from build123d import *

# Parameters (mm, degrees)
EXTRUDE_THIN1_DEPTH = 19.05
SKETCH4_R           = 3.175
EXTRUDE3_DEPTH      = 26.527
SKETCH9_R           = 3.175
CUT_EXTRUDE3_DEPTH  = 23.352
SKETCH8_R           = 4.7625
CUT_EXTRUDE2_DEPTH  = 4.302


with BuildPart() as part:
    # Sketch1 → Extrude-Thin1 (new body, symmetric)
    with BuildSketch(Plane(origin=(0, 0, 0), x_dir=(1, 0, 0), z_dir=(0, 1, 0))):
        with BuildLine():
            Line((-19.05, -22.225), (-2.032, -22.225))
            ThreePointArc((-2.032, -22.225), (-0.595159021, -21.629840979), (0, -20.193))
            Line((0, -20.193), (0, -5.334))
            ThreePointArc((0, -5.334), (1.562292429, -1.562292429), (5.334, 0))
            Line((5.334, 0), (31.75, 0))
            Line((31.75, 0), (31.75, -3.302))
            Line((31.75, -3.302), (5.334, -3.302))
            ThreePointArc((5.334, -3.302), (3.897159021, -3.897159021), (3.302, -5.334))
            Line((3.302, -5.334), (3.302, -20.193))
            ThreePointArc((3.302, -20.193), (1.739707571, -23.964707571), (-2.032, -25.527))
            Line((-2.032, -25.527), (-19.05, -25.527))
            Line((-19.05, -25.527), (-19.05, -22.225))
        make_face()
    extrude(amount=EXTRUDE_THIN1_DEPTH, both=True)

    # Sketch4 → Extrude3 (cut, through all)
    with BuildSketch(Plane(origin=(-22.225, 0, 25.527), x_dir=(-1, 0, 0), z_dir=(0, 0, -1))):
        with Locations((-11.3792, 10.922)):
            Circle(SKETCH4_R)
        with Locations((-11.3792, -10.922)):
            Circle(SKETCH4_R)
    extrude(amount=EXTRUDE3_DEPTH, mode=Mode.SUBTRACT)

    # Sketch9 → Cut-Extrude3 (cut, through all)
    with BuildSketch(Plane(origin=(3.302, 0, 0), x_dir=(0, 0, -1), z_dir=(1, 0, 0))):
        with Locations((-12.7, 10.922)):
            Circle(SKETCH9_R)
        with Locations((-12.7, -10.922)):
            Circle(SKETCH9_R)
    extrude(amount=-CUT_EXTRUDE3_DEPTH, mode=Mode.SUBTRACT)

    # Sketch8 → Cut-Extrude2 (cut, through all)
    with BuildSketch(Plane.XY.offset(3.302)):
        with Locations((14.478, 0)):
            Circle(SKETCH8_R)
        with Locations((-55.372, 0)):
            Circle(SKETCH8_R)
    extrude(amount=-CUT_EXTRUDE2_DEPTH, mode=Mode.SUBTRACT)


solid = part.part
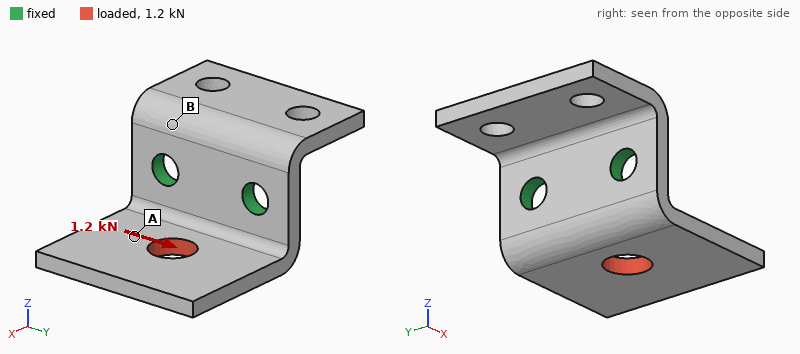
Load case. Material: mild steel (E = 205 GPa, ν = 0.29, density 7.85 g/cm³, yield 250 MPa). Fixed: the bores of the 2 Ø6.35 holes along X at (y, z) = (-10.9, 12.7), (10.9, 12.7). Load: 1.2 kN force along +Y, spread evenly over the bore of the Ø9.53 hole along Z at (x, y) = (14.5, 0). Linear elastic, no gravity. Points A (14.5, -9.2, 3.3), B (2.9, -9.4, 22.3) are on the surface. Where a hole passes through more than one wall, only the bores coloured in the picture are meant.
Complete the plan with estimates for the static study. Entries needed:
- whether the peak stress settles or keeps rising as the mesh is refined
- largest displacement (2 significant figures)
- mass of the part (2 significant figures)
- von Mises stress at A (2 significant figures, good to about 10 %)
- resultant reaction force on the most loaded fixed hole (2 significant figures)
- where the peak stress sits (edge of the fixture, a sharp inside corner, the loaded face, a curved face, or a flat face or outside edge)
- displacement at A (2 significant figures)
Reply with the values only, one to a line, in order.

keeps rising
37 µm
64 g
33 MPa
960 N
edge of the fixture
17 µm
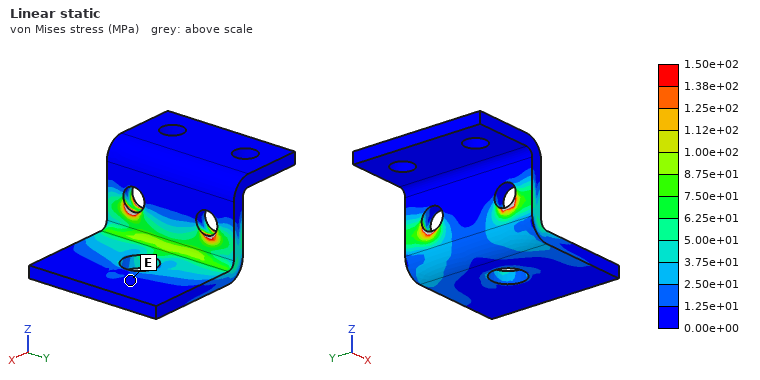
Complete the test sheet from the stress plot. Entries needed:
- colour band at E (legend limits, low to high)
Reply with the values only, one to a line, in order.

0.00e+00 to 1.25e+01 MPa
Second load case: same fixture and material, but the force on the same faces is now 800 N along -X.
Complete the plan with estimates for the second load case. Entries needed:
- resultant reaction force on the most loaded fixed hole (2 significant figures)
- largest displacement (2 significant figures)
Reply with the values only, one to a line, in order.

400 N
47 µm
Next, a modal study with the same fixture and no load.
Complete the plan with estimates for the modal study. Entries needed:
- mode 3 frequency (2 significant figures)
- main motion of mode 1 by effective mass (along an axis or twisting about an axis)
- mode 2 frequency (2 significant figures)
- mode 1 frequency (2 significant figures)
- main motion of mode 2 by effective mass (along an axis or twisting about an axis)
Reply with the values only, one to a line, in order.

4600 Hz
along Z
4000 Hz
2100 Hz
along Z
